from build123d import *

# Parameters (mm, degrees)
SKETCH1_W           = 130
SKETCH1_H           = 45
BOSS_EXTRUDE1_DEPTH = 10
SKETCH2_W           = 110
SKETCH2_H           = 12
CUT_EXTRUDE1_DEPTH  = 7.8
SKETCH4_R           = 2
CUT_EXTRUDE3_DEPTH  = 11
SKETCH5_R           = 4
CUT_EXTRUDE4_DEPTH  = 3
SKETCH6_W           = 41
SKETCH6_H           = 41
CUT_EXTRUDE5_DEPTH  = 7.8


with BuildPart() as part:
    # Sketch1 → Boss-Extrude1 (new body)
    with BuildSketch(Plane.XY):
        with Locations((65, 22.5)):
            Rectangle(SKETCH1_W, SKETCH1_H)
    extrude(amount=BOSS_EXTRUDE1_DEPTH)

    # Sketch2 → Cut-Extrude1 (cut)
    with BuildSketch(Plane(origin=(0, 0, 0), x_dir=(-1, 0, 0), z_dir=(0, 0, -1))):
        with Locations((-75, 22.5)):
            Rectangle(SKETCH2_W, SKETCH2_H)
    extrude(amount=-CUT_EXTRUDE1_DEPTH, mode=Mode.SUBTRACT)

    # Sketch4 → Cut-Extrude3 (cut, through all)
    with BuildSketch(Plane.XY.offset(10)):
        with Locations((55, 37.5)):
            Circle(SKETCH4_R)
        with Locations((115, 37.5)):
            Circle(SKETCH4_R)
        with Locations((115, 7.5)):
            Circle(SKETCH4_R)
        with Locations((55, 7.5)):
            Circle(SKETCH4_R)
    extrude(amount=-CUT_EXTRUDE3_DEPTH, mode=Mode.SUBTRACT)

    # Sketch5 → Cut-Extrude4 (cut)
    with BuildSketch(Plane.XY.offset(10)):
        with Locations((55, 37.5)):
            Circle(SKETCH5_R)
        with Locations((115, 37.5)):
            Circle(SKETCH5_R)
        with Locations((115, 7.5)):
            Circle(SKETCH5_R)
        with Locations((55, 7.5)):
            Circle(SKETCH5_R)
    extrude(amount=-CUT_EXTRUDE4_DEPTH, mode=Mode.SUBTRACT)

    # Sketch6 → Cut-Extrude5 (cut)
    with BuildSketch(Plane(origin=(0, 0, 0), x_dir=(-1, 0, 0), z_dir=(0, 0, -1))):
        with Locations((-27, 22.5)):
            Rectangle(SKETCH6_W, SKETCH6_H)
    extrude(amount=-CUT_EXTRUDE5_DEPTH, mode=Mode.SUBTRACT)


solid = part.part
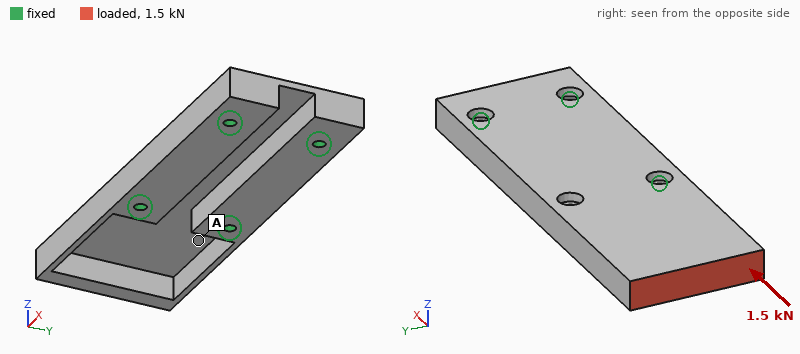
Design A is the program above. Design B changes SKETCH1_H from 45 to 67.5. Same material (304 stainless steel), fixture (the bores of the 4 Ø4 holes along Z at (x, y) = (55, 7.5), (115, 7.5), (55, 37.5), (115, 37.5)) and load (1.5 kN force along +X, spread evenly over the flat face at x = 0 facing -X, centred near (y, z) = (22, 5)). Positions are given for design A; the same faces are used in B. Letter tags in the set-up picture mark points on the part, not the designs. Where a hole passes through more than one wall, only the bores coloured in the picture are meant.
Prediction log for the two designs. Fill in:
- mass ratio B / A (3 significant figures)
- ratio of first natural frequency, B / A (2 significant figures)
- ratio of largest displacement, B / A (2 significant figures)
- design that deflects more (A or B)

1.80
1.2
0.20
A
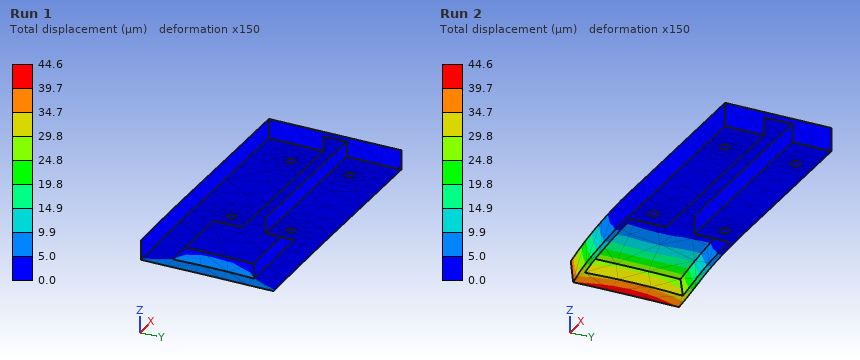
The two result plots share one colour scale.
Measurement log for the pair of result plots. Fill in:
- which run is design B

Run 1
